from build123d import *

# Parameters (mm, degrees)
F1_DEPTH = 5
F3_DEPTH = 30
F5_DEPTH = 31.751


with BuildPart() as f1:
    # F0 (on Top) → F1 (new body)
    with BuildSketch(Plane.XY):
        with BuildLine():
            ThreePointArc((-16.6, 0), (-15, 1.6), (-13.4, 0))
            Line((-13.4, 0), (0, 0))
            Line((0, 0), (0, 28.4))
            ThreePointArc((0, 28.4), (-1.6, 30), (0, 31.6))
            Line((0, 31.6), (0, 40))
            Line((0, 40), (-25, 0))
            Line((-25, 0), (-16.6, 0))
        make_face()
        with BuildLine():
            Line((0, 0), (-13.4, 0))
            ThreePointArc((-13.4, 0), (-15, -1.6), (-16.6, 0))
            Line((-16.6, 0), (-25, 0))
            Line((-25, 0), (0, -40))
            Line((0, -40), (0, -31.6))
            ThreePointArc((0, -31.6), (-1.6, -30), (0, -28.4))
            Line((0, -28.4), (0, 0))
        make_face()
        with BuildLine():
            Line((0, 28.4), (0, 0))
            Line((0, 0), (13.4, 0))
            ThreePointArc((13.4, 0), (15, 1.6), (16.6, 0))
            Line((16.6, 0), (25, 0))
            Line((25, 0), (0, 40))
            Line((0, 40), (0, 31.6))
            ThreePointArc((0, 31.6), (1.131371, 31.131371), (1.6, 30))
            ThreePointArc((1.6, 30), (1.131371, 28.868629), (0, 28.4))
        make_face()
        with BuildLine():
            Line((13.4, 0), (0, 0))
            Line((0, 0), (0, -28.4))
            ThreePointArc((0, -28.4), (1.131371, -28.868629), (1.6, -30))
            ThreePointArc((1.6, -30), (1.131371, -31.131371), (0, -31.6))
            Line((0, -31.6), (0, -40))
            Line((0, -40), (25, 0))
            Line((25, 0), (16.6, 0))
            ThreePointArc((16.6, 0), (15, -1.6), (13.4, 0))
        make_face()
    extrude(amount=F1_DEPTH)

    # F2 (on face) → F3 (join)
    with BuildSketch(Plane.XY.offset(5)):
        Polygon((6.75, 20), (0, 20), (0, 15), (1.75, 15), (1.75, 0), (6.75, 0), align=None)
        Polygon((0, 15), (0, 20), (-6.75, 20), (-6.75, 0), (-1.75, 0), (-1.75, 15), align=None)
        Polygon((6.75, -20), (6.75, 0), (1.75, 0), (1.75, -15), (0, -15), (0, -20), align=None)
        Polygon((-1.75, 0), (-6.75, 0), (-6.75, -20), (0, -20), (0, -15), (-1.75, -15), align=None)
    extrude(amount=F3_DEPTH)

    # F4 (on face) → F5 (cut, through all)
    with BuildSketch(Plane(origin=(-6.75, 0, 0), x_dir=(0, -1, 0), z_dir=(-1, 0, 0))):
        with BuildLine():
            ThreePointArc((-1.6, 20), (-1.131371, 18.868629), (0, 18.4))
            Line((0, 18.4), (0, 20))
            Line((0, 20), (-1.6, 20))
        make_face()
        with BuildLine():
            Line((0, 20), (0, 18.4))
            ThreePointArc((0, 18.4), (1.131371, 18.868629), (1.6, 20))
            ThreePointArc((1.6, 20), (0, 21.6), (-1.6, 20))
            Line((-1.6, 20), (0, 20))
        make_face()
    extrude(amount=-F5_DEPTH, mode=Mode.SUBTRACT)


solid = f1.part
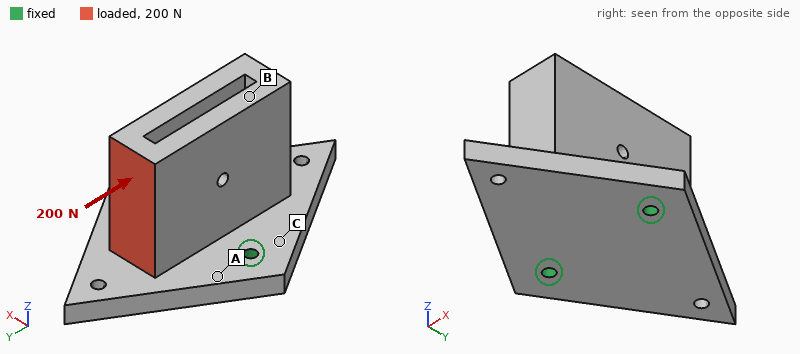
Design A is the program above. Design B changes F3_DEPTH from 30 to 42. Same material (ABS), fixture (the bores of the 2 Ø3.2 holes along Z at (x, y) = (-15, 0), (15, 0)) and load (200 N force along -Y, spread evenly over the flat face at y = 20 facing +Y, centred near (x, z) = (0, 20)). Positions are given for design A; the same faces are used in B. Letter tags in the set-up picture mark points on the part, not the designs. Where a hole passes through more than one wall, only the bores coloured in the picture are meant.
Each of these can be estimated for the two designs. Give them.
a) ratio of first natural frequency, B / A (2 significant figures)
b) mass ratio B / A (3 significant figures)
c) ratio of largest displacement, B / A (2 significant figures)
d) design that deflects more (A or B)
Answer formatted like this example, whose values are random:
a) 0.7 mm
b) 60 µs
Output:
a) 0.72
b) 1.23
c) 1.6
d) B
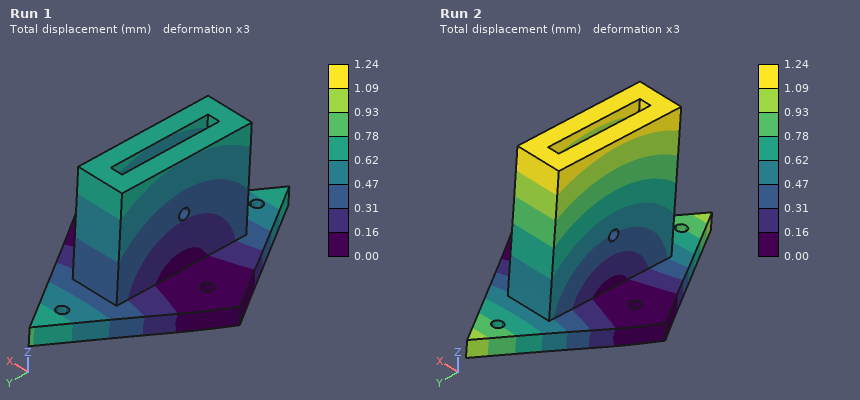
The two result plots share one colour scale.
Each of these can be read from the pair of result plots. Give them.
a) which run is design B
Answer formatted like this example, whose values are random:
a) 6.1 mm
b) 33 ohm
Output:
a) Run 2
